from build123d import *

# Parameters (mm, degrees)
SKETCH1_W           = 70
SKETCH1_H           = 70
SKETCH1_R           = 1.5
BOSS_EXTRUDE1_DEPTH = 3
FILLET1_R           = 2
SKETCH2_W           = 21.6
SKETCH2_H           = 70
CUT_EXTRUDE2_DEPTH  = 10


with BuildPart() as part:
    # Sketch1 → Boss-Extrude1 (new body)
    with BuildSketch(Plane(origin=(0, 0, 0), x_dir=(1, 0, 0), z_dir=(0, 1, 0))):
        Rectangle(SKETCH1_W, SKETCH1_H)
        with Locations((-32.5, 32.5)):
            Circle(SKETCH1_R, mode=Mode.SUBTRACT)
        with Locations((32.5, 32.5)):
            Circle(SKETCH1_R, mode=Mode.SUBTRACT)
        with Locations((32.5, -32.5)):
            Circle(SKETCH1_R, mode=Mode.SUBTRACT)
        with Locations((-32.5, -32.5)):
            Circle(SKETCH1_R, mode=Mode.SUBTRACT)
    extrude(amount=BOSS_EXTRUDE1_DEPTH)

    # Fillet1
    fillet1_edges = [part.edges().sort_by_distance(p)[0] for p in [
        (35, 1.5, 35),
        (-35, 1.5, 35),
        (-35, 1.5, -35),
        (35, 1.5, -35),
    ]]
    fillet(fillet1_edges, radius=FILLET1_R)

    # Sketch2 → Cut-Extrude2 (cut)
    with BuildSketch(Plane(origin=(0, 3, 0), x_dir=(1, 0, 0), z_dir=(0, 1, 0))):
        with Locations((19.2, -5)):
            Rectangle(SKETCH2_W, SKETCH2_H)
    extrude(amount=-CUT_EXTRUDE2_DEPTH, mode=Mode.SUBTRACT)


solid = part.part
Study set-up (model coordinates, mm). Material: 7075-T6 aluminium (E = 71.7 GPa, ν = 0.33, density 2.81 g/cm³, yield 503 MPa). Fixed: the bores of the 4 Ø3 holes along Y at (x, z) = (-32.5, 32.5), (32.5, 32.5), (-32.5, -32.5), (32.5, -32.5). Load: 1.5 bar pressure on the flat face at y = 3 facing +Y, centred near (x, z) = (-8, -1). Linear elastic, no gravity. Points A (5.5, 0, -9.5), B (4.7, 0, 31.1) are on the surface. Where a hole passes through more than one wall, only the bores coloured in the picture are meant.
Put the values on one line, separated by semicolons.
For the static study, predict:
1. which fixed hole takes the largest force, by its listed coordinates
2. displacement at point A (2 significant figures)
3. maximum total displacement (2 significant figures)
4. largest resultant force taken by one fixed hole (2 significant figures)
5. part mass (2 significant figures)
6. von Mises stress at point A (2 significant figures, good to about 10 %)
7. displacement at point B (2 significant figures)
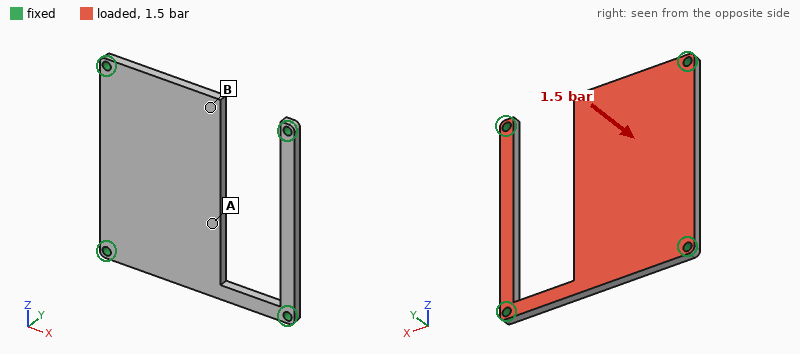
(-32.5, 32.5); 0.36 mm; 0.49 mm; 220 N; 29 g; 41 MPa; 0.43 mm
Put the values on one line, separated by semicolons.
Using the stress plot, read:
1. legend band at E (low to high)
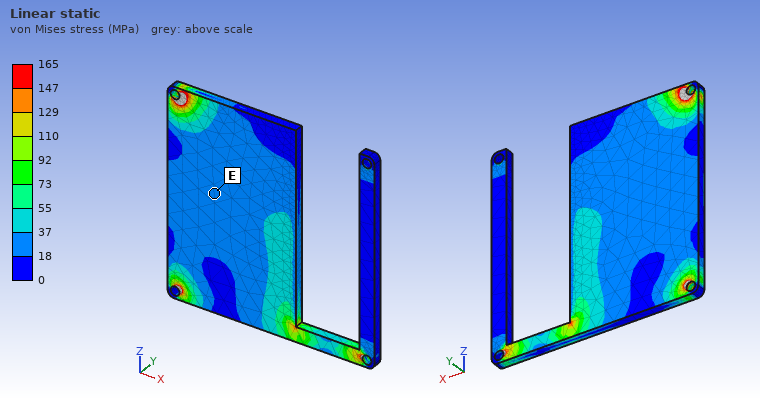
18 to 37 MPa
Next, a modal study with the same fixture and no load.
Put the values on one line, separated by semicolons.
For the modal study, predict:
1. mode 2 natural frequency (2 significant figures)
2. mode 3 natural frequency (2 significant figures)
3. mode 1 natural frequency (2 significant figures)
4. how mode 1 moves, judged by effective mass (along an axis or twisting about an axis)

2800 Hz; 3800 Hz; 1300 Hz; along Y
